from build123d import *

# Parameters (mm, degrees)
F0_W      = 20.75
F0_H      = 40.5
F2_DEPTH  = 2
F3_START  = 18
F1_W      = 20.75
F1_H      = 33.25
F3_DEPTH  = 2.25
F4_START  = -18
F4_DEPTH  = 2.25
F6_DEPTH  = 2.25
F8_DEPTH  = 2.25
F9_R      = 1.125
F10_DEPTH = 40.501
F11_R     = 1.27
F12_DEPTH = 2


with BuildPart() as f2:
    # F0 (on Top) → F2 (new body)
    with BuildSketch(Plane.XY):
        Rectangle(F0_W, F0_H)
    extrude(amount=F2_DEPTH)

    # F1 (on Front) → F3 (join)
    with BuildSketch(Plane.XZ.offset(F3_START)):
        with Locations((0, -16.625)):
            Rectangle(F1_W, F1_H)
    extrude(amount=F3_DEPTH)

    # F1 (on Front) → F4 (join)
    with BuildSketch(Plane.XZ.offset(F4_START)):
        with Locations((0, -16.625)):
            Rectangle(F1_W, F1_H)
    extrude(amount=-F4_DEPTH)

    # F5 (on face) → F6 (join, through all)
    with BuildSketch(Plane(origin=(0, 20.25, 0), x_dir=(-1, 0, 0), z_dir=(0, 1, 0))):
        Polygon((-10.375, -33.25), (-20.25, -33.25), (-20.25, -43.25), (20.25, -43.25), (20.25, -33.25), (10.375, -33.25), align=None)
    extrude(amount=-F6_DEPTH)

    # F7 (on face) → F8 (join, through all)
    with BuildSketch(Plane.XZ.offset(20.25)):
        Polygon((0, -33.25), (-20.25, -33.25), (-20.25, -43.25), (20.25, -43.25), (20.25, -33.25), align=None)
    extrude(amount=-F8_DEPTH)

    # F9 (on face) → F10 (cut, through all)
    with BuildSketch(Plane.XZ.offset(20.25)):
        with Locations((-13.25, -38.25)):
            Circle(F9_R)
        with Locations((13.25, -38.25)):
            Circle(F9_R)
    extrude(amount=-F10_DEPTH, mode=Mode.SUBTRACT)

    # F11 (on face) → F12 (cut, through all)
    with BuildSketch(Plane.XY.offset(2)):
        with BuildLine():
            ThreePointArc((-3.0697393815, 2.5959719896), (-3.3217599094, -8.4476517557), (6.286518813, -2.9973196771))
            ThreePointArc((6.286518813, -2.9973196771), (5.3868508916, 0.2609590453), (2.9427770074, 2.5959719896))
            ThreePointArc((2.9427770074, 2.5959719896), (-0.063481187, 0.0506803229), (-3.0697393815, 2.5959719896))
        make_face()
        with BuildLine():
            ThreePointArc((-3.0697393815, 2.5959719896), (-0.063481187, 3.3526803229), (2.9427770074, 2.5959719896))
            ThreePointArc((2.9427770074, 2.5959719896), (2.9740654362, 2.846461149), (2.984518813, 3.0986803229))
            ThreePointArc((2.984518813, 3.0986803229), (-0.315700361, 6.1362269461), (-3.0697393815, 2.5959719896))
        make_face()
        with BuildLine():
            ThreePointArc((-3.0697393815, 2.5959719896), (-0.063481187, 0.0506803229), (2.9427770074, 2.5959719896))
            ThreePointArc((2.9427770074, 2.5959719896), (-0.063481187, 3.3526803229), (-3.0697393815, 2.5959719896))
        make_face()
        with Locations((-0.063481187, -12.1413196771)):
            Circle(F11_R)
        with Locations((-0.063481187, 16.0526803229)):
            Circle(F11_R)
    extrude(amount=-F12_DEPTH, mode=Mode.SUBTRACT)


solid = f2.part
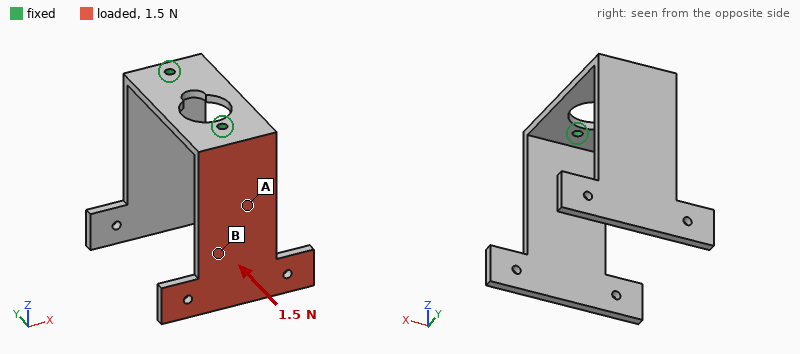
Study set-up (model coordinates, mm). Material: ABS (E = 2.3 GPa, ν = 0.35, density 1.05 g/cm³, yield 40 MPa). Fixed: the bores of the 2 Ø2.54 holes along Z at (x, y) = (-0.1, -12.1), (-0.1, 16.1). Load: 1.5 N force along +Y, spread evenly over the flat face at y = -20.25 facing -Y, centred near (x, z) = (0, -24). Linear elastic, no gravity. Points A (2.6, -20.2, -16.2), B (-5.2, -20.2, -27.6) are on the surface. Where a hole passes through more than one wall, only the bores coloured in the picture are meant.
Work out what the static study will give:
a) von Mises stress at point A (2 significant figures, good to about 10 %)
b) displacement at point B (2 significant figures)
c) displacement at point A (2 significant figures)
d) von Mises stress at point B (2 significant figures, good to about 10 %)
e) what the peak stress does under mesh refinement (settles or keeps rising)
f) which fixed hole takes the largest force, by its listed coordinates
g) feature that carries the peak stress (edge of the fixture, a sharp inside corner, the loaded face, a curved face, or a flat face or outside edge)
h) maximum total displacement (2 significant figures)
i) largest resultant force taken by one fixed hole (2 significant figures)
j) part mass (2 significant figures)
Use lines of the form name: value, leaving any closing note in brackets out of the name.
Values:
von Mises stress at point A: 0.85 MPa
displacement at point B: 0.44 mm
displacement at point A: 0.23 mm
von Mises stress at point B: 0.35 MPa
what the peak stress does under mesh refinement: keeps rising
which fixed hole takes the largest force, by its listed coordinates: (-0.1, -12.1)
feature that carries the peak stress: edge of the fixture
maximum total displacement: 0.76 mm
largest resultant force taken by one fixed hole: 1.5 N
part mass: 6.6 g
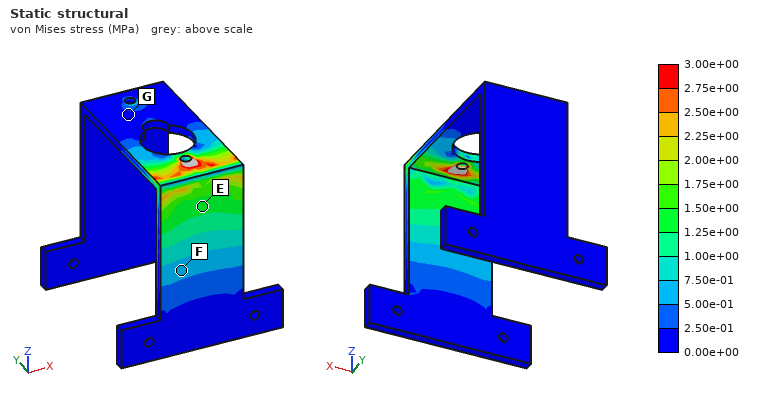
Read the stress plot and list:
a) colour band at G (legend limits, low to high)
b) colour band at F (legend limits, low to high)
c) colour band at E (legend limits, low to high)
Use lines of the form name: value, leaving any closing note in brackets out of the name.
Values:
colour band at G: 0.00e+00 to 2.50e-01 MPa
colour band at F: 5.00e-01 to 7.50e-01 MPa
colour band at E: 1.25e+00 to 1.50e+00 MPa
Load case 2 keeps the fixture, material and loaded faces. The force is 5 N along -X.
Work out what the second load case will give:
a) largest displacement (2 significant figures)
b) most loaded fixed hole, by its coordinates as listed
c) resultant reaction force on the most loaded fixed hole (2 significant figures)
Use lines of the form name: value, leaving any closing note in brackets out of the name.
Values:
largest displacement: 0.83 mm
most loaded fixed hole, by its coordinates as listed: (-0.1, -12.1)
resultant reaction force on the most loaded fixed hole: 6.0 N
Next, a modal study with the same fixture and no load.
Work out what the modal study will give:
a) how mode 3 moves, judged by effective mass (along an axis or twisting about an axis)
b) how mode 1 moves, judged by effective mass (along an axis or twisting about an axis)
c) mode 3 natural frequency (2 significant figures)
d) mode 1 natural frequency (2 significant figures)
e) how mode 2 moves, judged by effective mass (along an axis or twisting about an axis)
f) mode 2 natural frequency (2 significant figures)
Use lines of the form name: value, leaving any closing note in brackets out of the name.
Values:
how mode 3 moves, judged by effective mass: along X
how mode 1 moves, judged by effective mass: along Y
mode 3 natural frequency: 280 Hz
mode 1 natural frequency: 160 Hz
how mode 2 moves, judged by effective mass: along Y
mode 2 natural frequency: 190 Hz
